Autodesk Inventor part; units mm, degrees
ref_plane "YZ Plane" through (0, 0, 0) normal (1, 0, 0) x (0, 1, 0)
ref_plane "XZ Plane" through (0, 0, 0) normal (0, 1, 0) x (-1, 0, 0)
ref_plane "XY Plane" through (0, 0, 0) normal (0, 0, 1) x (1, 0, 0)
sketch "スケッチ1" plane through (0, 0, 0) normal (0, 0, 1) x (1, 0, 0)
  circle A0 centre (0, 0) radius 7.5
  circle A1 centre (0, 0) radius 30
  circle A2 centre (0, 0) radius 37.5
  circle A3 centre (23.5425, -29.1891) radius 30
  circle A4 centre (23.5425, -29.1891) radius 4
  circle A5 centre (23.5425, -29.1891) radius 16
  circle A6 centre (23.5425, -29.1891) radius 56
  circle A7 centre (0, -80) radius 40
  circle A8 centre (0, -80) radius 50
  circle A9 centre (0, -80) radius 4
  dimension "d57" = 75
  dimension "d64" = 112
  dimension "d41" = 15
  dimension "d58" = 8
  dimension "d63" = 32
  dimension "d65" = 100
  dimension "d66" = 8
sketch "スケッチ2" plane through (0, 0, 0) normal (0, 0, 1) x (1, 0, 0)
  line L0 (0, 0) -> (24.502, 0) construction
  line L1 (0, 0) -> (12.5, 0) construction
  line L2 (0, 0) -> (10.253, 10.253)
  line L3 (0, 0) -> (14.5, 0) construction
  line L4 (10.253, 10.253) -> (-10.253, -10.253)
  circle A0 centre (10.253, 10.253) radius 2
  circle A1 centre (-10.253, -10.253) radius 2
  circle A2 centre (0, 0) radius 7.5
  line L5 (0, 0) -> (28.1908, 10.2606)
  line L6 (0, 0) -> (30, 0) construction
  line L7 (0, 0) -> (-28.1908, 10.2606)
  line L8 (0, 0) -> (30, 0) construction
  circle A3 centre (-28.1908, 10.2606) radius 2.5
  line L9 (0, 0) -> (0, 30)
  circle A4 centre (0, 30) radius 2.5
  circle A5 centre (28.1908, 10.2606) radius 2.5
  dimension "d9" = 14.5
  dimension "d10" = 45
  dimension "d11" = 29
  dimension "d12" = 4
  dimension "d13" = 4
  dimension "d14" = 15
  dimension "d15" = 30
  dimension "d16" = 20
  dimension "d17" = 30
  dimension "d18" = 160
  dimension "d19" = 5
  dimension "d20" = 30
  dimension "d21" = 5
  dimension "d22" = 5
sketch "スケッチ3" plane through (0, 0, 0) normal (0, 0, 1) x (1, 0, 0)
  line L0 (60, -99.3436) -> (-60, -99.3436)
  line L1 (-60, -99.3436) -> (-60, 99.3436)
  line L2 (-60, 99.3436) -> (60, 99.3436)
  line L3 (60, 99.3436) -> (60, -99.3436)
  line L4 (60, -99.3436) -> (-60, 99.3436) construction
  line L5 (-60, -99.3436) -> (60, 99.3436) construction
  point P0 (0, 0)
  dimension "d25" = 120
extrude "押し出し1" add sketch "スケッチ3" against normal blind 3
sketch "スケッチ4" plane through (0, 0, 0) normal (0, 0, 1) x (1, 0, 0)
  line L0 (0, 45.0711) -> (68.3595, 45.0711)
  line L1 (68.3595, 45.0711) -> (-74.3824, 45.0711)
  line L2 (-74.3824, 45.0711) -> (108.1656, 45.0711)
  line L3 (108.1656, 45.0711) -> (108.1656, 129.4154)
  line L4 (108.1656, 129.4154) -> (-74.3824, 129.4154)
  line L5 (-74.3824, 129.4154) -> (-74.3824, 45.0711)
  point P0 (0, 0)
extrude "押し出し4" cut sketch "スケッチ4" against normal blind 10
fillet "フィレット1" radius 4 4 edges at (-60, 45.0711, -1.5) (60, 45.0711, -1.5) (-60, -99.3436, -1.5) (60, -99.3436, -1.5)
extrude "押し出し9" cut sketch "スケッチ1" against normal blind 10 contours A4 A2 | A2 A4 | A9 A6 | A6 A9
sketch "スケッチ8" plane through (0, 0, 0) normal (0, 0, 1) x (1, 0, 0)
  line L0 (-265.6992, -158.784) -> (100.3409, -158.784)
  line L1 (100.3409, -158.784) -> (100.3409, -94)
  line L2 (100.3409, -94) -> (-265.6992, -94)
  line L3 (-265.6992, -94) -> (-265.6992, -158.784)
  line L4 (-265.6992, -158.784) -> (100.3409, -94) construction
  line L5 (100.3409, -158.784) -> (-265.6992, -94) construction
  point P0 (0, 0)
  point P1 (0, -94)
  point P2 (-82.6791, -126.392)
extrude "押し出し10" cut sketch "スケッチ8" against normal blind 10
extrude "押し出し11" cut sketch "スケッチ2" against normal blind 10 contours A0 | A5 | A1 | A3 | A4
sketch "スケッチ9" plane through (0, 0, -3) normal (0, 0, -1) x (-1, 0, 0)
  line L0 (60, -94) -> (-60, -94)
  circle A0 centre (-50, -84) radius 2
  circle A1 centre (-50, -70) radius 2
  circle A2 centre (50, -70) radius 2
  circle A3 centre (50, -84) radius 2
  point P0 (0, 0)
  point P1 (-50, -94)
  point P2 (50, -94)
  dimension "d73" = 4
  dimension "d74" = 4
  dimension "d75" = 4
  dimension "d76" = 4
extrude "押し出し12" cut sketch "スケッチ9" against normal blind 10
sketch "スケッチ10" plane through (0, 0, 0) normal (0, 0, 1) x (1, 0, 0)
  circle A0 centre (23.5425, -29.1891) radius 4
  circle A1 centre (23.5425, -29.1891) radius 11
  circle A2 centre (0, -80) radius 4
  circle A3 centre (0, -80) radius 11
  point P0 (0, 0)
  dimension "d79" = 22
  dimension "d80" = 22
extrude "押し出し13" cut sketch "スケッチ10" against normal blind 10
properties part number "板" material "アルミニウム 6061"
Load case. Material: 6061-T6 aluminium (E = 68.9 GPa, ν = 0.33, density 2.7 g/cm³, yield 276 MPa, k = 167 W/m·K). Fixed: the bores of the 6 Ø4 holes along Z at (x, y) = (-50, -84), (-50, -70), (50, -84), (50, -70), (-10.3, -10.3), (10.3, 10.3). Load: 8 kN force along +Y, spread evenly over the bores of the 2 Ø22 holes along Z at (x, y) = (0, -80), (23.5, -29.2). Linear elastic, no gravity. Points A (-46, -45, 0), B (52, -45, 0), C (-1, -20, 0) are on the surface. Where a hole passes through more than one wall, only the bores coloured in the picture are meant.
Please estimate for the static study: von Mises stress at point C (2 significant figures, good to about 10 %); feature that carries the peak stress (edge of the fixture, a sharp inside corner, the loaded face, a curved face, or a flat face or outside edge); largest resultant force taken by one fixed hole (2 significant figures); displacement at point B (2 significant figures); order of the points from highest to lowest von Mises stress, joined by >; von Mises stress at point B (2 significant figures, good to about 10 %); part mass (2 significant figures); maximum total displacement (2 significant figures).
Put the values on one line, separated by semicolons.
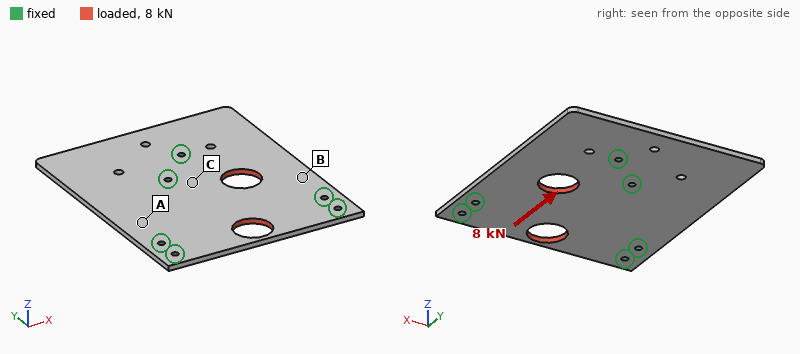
31 MPa; a flat face or outside edge; 2.1 kN; 12 µm; C > B > A; 17 MPa; 130 g; 59 µm
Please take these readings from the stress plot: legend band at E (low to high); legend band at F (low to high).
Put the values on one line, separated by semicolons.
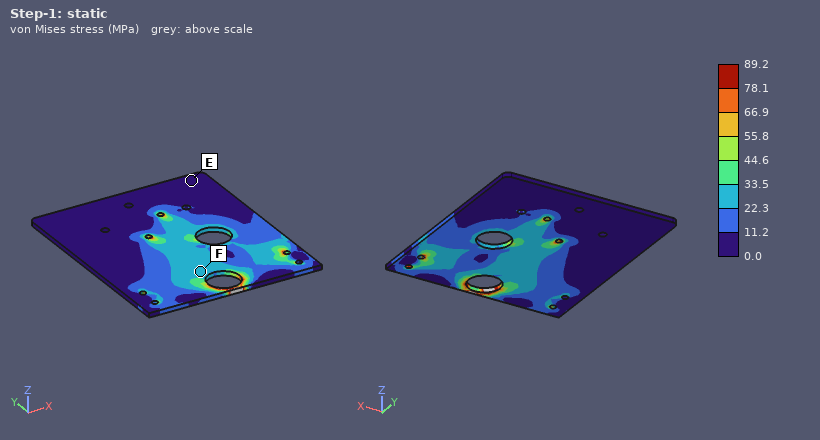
0.0 to 11.2 MPa; 22.3 to 33.5 MPa
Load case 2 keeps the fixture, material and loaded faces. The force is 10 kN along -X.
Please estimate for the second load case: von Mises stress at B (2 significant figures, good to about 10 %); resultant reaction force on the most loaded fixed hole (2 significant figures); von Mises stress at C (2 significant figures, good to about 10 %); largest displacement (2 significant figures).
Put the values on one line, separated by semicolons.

16 MPa; 2.3 kN; 26 MPa; 29 µm
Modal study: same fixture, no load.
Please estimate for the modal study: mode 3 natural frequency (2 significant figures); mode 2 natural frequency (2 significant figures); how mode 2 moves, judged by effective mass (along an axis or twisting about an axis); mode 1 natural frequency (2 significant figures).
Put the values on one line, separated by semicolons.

1500 Hz; 970 Hz; along Z; 730 Hz
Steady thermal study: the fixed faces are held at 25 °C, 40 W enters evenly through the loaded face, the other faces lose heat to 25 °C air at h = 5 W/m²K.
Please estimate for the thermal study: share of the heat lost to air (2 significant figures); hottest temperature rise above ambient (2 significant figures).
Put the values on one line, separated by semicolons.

3.3 %; 29 K
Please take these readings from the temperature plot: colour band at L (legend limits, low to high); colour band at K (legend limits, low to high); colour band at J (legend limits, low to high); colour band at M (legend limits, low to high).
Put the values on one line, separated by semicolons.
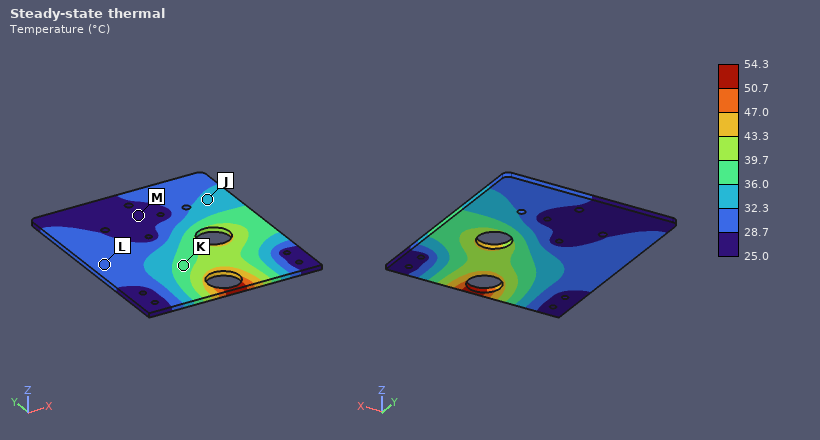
28.7 to 32.3 °C; 36.0 to 39.7 °C; 32.3 to 36.0 °C; 25.0 to 28.7 °C
